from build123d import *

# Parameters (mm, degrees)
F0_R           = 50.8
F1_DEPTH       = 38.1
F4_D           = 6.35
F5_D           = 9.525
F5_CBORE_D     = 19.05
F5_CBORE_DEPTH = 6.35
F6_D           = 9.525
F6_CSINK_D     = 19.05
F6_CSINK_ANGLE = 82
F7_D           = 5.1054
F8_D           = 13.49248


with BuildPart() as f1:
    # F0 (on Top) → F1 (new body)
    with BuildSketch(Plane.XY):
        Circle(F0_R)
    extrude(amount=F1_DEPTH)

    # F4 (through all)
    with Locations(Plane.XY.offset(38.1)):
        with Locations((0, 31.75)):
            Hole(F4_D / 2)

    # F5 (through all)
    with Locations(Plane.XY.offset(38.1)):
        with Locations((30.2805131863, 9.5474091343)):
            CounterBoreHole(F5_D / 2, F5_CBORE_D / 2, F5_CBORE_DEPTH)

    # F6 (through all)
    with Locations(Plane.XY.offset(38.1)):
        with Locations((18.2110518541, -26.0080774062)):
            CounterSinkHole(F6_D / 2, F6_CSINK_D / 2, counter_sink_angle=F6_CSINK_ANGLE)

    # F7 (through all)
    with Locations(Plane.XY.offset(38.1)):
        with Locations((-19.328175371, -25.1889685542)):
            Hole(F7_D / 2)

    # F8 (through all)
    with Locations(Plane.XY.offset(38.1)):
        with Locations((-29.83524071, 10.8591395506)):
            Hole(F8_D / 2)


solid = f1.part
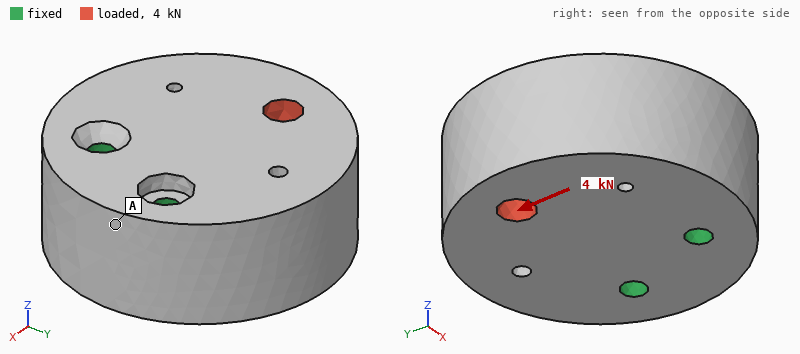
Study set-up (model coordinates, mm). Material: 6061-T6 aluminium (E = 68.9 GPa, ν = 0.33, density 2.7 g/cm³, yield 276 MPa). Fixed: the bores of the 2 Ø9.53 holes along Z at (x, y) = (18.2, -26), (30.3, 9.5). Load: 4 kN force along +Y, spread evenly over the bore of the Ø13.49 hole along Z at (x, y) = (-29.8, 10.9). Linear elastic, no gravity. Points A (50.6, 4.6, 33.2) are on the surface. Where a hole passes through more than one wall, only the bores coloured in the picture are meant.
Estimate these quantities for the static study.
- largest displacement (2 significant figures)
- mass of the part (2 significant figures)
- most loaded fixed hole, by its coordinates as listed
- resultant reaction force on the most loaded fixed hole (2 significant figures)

9.2 µm
790 g
(18.2, -26)
5.8 kN
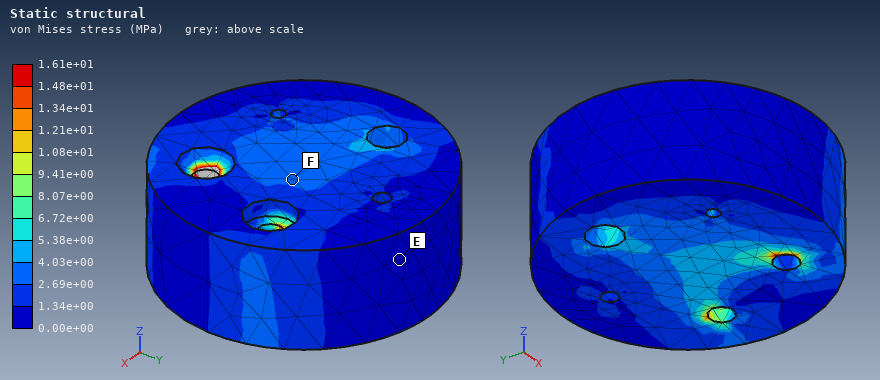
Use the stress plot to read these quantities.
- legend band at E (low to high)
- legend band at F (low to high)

0.00e+00 to 1.34e+00 MPa
2.69e+00 to 4.03e+00 MPa
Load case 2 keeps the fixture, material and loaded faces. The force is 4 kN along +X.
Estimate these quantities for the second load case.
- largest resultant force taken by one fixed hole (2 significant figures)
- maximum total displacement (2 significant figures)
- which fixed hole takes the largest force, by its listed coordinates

3.7 kN
4.1 µm
(30.3, 9.5)
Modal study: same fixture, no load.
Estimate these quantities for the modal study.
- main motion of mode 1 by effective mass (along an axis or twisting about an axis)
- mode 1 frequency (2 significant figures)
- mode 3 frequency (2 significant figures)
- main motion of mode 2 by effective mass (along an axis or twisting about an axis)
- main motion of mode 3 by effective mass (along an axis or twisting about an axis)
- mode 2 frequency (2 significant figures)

along Z
4400 Hz
7900 Hz
along Y
twisting about X
6000 Hz
